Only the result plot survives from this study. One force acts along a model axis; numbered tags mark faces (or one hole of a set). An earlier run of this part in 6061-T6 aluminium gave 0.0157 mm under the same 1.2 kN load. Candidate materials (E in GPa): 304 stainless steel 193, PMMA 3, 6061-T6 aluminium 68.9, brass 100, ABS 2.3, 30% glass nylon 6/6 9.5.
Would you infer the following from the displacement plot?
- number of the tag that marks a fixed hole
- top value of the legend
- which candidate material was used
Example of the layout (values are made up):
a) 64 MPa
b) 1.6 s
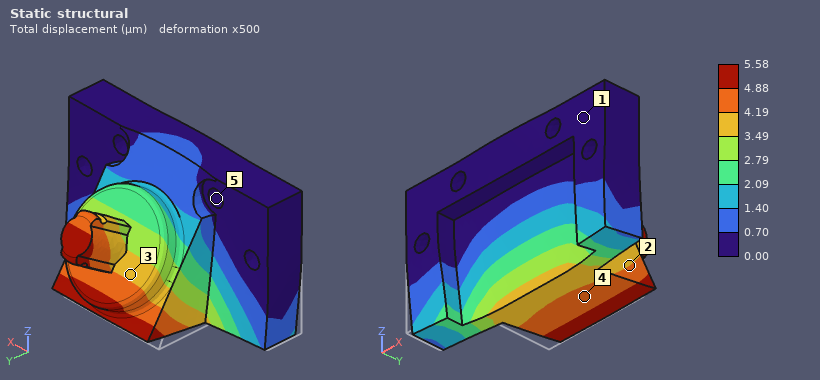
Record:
a) 5
b) 5.58 µm
c) 304 stainless steel
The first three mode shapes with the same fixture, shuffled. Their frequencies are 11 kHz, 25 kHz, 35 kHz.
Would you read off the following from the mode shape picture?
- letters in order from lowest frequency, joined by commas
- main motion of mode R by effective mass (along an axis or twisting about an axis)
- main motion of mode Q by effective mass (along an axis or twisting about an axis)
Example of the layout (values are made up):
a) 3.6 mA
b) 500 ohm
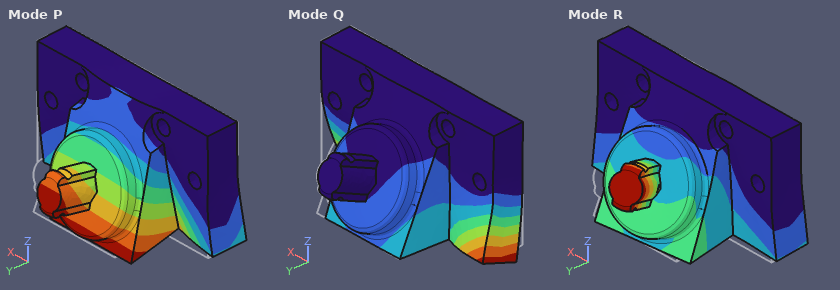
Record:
a) P, R, Q
b) along X
c) along X
